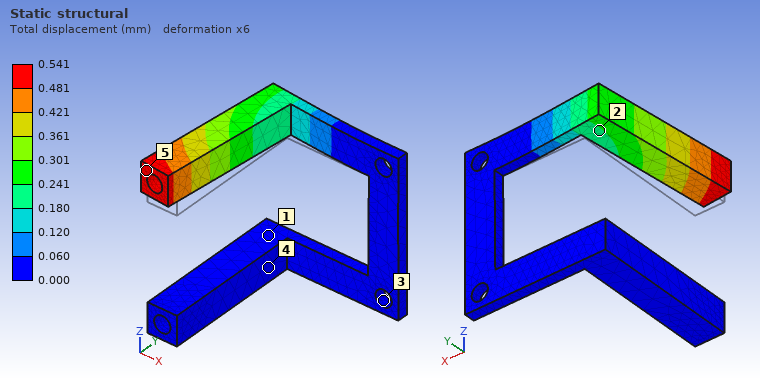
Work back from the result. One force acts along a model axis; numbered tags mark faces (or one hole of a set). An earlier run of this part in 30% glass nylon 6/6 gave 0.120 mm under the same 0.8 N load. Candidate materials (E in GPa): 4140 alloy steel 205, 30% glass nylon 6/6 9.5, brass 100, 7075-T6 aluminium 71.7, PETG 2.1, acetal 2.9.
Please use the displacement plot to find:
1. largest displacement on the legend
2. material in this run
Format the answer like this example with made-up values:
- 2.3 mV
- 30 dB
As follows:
- 0.541 mm
- PETG
